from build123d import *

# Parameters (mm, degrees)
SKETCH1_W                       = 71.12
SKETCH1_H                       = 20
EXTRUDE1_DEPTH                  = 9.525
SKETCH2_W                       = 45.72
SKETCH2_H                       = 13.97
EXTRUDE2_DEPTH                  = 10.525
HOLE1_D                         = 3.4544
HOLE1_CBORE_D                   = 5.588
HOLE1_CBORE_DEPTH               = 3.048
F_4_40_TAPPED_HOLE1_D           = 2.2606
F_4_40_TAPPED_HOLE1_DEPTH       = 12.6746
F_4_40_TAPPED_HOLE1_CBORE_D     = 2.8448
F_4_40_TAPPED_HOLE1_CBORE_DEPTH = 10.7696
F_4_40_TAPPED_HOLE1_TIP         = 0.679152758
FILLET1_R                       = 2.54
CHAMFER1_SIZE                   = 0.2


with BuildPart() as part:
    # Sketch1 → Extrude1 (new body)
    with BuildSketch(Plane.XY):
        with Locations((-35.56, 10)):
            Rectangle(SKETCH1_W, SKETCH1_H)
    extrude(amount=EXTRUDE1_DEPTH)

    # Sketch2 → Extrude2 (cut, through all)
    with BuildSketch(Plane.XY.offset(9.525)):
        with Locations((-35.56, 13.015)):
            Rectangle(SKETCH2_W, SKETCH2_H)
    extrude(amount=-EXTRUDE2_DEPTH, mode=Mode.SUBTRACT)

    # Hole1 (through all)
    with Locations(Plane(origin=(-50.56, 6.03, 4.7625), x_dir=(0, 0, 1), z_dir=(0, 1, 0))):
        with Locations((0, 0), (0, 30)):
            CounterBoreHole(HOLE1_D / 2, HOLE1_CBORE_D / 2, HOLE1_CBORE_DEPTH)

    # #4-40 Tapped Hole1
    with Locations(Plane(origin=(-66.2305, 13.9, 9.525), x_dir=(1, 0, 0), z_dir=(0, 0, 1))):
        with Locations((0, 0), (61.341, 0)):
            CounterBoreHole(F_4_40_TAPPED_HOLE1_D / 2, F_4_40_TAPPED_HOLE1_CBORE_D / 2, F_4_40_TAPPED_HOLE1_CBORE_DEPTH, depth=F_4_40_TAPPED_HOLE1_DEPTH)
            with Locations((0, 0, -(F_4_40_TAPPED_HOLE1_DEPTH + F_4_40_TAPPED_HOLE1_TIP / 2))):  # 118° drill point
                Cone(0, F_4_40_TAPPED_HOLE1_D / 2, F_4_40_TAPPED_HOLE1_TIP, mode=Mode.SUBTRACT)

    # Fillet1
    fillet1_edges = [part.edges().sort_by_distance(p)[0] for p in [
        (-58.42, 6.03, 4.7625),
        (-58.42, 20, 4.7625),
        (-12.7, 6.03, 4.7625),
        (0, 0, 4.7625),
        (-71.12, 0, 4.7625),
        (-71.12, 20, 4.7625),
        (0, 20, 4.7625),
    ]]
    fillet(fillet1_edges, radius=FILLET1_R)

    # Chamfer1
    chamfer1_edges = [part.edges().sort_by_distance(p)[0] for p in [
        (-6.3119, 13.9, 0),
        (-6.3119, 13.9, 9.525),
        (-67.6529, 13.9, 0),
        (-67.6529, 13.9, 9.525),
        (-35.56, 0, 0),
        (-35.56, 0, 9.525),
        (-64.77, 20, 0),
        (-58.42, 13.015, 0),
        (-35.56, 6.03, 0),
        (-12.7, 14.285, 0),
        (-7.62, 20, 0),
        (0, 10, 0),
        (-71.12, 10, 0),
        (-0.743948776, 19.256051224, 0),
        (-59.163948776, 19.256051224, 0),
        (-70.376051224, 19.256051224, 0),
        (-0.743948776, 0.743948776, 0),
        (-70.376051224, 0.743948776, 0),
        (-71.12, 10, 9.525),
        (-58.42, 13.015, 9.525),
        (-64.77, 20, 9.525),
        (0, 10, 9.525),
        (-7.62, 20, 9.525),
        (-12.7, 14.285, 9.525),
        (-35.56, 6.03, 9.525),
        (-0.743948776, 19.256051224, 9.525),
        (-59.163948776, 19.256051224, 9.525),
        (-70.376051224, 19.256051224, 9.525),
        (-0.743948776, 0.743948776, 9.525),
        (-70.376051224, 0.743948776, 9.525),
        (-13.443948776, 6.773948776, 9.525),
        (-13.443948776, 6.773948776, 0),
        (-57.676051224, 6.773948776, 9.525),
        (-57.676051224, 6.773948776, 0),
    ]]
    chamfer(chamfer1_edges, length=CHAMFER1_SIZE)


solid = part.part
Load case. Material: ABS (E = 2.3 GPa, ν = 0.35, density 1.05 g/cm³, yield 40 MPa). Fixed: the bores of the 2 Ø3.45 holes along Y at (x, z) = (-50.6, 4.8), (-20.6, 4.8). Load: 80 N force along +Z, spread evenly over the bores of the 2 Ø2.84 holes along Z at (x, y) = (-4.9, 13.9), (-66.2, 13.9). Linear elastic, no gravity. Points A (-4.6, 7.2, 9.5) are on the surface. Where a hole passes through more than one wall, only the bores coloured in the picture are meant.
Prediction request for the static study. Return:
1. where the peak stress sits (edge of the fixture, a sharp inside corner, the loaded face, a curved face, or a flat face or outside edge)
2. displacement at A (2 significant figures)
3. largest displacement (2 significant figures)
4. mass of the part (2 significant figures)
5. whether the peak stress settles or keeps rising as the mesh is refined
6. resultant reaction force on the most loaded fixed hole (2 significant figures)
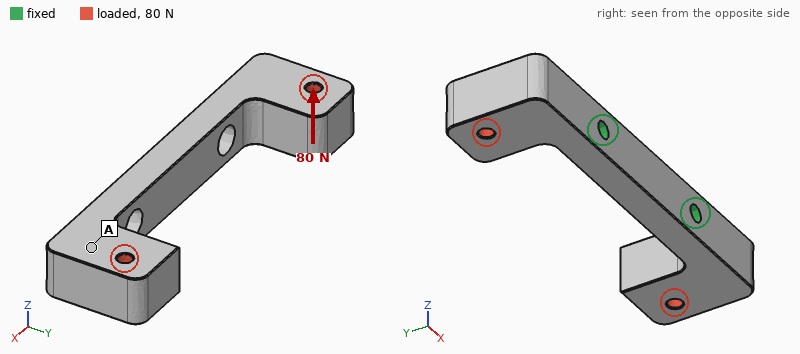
edge of the fixture
0.20 mm
0.42 mm
7.4 g
keeps rising
40 N
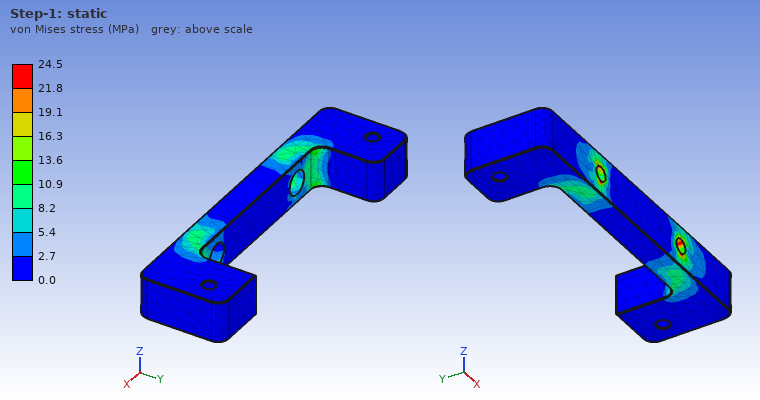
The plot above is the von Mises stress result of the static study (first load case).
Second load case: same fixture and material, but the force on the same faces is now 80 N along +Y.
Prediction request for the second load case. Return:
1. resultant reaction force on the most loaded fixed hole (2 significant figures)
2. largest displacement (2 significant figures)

69 N
0.42 mm
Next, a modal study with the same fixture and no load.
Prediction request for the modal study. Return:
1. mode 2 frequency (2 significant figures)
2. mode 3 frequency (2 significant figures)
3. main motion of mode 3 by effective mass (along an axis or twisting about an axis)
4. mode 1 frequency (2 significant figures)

1200 Hz
1400 Hz
along Z
1100 Hz
